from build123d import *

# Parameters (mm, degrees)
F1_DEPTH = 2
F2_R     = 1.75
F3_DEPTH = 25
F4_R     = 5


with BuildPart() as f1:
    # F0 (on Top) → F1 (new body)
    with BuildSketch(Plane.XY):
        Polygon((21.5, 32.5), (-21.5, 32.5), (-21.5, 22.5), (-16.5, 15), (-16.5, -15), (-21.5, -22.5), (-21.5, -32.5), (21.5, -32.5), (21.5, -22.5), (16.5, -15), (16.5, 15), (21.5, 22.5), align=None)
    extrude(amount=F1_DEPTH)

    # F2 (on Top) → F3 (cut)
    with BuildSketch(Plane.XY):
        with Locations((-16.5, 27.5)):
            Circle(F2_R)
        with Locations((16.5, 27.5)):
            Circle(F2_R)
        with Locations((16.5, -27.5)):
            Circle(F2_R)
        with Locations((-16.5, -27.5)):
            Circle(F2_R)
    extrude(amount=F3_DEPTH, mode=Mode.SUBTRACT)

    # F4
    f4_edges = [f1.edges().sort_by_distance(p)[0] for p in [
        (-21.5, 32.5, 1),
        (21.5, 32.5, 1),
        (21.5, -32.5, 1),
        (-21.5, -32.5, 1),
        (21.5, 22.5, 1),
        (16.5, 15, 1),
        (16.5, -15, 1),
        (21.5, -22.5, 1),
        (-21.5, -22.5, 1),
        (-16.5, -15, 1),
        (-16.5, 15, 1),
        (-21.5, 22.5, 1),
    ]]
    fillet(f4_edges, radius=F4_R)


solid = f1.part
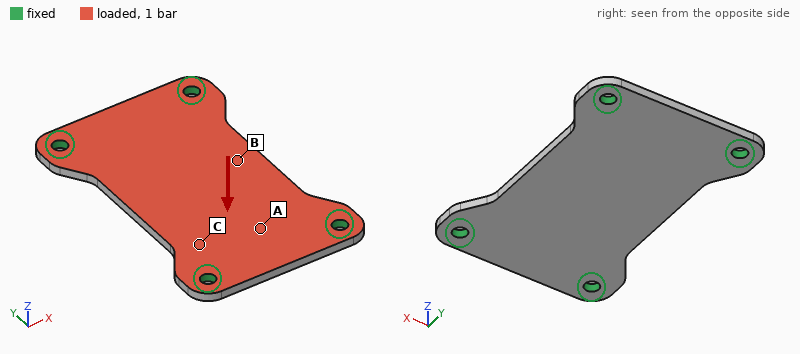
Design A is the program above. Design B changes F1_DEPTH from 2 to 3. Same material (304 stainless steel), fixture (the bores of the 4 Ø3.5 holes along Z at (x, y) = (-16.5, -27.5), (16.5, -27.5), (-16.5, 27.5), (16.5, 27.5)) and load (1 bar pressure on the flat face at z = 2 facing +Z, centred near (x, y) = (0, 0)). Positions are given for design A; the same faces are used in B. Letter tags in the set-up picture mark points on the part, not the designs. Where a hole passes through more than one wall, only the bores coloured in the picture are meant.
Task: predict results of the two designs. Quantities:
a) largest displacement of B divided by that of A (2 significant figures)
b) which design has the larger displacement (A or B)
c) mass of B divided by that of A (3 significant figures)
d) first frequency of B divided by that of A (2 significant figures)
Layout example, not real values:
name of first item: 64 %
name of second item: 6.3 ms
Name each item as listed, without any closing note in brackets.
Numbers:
largest displacement of B divided by that of A: 0.31
which design has the larger displacement: A
mass of B divided by that of A: 1.50
first frequency of B divided by that of A: 1.5
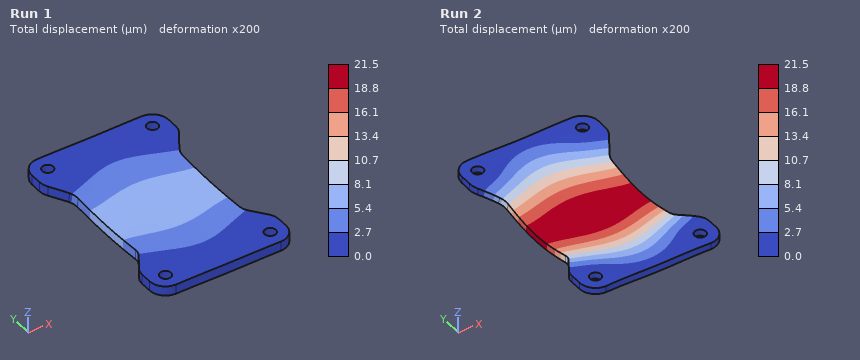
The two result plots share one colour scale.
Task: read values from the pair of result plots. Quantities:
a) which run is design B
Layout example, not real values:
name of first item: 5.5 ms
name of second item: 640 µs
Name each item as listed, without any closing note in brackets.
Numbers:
which run is design B: Run 1
